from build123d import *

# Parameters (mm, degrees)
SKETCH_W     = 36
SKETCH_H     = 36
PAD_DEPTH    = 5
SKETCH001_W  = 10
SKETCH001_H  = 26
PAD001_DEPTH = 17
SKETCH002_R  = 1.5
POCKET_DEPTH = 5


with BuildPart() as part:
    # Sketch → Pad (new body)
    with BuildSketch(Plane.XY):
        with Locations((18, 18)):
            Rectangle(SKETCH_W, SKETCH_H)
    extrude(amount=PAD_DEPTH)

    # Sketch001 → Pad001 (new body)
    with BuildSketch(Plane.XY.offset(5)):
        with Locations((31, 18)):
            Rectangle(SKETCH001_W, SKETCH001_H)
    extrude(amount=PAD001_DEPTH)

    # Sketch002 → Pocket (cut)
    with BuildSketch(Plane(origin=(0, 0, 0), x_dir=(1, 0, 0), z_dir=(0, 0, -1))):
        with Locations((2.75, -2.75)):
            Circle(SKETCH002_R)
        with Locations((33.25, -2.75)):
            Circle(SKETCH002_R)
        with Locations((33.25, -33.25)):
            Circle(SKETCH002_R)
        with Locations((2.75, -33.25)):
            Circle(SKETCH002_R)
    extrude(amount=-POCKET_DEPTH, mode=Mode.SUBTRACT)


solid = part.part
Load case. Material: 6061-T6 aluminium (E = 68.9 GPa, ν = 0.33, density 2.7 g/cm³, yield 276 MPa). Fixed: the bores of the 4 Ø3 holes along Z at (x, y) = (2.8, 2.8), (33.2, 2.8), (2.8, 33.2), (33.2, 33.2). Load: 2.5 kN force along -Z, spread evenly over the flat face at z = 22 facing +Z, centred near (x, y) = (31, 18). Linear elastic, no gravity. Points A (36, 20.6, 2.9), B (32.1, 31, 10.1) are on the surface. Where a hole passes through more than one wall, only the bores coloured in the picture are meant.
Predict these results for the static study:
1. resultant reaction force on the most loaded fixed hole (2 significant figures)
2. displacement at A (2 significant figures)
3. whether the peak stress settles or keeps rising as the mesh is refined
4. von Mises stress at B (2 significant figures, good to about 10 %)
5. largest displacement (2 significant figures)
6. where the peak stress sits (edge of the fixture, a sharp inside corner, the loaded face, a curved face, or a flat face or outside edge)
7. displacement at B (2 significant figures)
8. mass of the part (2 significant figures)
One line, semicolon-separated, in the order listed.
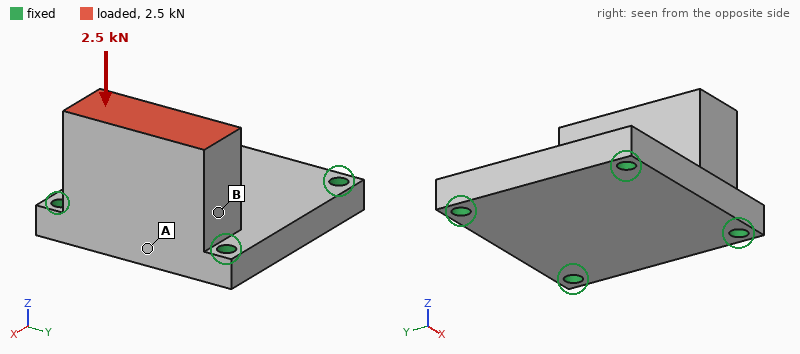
1.3 kN; 7.3 µm; keeps rising; 21 MPa; 11 µm; edge of the fixture; 6.8 µm; 29 g
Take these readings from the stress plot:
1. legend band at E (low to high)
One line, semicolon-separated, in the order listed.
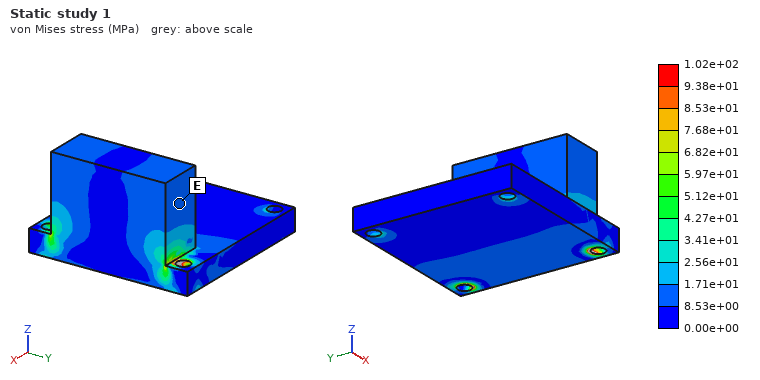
8.53e+00 to 1.71e+01 MPa
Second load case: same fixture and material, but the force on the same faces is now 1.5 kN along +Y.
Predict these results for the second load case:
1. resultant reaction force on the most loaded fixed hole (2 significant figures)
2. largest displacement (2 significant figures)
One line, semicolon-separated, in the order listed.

1.2 kN; 16 µm
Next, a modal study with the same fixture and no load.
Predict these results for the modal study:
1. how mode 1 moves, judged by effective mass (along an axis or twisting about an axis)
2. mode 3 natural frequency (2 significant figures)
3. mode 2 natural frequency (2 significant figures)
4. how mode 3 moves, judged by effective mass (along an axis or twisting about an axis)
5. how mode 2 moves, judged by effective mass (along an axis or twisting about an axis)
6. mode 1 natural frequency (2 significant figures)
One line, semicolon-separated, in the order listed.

along X; 22 kHz; 20 kHz; along Y; along Z; 9100 Hz
